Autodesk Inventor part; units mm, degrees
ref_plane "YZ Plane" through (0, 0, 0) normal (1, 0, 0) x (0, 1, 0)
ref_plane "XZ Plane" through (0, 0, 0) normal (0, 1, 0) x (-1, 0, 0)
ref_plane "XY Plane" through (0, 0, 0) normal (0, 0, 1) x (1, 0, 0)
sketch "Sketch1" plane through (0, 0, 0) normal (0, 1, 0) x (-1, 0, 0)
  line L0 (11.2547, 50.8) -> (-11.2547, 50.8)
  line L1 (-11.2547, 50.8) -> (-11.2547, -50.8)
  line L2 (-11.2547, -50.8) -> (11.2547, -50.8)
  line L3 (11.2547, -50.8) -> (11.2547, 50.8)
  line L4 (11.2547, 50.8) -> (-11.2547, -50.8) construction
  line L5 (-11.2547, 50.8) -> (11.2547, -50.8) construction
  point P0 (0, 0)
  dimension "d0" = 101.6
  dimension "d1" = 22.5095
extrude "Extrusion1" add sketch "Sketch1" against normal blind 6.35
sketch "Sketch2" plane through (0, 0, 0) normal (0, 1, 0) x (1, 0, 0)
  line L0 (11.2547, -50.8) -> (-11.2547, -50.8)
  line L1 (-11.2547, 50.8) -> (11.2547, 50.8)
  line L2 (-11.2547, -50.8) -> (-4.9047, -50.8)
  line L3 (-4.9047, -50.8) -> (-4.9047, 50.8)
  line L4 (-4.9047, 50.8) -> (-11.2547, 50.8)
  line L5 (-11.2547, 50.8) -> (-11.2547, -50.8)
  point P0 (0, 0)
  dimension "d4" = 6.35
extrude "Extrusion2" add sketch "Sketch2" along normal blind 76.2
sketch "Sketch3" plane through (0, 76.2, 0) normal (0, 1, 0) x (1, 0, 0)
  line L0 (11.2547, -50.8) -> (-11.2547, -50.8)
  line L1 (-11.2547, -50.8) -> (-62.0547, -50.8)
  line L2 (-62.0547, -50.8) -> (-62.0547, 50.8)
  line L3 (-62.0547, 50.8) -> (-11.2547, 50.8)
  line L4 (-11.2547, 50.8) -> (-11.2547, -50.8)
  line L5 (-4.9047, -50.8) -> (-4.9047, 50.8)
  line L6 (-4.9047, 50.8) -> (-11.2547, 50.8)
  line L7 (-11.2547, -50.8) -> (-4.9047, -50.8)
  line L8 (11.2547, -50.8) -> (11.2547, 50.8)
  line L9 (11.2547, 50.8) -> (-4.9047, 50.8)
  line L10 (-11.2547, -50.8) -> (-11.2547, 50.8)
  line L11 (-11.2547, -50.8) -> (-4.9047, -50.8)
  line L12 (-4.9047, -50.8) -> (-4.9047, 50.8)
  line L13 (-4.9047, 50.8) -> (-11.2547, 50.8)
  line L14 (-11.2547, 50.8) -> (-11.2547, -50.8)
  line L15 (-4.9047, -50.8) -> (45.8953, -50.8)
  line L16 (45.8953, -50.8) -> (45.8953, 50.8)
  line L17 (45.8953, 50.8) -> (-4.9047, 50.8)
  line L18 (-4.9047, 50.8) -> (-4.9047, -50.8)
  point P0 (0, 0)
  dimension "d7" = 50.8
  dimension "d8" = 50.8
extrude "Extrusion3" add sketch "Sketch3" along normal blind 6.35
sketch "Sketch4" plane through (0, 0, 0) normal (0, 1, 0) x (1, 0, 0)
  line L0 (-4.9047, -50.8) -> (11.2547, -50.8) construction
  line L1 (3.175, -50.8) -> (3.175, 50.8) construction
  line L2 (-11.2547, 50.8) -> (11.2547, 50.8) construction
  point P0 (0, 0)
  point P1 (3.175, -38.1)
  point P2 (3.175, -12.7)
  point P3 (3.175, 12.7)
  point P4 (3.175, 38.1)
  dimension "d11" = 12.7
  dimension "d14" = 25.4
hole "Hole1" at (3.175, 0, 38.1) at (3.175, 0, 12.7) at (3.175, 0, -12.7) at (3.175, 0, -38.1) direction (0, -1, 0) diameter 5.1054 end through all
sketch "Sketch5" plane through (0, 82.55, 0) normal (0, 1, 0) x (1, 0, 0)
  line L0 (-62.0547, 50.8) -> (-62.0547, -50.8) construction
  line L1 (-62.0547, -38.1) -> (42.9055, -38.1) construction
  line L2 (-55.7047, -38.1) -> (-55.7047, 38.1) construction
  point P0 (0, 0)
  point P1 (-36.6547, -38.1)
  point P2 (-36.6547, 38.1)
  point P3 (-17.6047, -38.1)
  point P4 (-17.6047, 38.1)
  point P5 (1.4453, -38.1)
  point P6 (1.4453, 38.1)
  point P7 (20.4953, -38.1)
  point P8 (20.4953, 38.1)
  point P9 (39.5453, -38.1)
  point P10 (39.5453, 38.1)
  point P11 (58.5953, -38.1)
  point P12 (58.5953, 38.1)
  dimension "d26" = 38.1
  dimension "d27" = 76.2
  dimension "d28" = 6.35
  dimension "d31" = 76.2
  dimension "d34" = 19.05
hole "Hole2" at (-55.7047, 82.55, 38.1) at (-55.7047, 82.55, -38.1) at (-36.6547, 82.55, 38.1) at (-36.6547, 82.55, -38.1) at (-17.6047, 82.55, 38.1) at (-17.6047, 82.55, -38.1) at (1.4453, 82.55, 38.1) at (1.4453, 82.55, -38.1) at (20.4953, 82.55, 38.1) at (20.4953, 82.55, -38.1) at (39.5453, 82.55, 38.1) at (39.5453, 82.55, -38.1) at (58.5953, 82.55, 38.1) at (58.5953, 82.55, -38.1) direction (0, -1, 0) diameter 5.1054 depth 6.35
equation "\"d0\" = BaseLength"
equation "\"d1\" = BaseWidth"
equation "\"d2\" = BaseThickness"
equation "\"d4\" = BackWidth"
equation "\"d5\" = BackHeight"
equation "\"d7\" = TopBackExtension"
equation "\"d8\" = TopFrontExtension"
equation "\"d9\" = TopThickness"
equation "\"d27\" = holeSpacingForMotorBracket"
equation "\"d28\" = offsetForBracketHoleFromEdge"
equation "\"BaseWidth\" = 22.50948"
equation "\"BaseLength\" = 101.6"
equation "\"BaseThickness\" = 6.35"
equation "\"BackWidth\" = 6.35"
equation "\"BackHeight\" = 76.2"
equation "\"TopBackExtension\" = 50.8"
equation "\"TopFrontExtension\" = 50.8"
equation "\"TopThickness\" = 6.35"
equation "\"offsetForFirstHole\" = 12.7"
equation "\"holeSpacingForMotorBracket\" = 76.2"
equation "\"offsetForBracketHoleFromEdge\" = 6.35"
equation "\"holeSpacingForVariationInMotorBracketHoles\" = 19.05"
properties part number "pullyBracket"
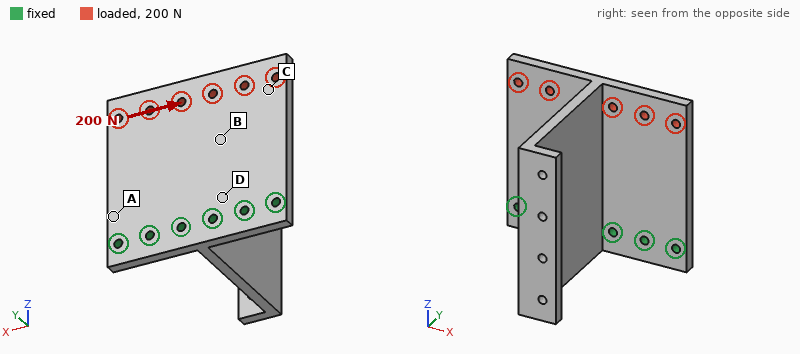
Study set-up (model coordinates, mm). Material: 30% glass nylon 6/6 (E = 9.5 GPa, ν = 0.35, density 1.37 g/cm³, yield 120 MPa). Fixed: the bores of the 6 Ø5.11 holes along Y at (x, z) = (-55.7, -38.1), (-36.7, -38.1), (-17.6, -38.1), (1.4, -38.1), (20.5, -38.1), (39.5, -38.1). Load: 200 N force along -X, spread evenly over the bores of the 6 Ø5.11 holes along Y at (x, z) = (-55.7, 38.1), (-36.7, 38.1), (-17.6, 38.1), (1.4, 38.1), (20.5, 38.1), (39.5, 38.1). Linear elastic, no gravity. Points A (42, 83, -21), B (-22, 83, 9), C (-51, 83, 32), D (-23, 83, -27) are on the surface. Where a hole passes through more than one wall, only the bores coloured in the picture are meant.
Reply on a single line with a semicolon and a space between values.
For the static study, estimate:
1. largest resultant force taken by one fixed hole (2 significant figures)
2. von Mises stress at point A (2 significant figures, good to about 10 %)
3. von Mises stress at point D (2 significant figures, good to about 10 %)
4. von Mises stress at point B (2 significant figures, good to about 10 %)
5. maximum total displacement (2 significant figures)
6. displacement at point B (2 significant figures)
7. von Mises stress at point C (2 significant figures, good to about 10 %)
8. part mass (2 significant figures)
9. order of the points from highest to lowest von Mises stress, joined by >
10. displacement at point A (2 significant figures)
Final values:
120 N; 0.97 MPa; 0.59 MPa; 0.74 MPa; 15 µm; 6.5 µm; 0.46 MPa; 180 g; A > B > D > C; 3.1 µm
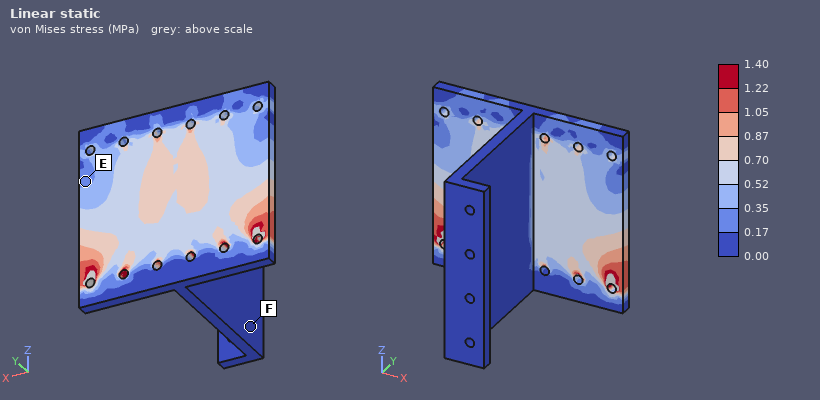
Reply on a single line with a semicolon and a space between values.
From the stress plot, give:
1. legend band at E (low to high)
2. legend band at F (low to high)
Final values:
0.17 to 0.35 MPa; 0.00 to 0.17 MPa
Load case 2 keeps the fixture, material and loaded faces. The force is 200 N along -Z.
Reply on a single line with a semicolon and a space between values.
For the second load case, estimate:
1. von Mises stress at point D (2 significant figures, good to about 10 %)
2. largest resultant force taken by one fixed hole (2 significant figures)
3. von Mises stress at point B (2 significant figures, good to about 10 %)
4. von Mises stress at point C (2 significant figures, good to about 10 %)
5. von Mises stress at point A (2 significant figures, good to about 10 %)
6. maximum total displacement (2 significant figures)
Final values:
0.25 MPa; 36 N; 0.26 MPa; 0.31 MPa; 0.29 MPa; 2.9 µm
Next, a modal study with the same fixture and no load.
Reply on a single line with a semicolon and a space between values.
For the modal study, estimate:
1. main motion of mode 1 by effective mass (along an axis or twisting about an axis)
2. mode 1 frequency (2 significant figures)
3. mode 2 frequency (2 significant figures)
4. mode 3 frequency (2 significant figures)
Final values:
along X; 250 Hz; 330 Hz; 610 Hz
